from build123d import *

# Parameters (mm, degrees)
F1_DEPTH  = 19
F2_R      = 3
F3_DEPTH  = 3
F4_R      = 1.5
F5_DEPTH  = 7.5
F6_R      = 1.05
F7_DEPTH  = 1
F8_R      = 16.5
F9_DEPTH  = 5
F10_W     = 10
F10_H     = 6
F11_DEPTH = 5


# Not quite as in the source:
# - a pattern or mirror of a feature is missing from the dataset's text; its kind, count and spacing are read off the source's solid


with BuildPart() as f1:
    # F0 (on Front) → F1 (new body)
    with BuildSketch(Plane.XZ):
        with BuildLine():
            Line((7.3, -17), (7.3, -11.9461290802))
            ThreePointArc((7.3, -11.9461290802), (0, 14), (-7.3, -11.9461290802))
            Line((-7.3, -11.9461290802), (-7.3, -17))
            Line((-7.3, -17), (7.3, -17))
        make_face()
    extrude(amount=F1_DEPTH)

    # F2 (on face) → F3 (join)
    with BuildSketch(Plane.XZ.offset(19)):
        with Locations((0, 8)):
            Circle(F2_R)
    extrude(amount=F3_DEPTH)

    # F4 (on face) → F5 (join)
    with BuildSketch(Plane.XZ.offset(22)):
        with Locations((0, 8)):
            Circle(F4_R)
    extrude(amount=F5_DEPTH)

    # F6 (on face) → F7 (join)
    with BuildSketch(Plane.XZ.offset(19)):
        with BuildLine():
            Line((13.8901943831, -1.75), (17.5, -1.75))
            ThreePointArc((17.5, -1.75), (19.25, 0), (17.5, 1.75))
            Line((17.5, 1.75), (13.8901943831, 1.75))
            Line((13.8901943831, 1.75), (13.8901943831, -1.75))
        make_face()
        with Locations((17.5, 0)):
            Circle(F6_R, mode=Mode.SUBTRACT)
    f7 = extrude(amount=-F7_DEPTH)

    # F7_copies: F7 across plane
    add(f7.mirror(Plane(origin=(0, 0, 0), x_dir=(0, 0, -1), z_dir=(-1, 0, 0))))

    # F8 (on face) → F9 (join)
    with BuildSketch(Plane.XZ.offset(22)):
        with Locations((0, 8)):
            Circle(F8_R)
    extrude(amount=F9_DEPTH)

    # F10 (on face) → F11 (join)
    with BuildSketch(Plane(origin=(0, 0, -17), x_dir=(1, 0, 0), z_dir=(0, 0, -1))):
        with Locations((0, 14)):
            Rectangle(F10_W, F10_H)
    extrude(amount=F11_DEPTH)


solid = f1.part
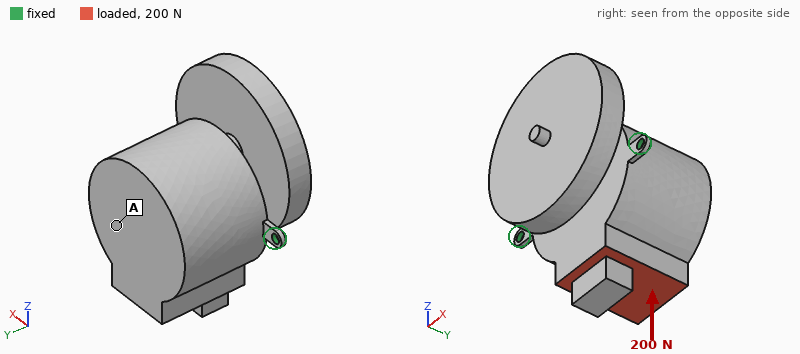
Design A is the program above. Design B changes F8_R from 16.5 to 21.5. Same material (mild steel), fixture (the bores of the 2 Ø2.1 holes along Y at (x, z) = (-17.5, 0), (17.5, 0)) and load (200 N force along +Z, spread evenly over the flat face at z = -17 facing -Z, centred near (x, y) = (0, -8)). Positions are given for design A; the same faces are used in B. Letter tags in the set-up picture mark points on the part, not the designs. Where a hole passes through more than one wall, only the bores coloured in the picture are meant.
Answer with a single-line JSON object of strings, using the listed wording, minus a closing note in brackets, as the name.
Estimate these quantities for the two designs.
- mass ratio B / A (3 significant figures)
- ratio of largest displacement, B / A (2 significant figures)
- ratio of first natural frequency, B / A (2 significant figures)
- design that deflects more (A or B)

{"mass ratio B / A": "1.17", "ratio of largest displacement, B / A": "1.2", "ratio of first natural frequency, B / A": "0.88", "design that deflects more": "B"}
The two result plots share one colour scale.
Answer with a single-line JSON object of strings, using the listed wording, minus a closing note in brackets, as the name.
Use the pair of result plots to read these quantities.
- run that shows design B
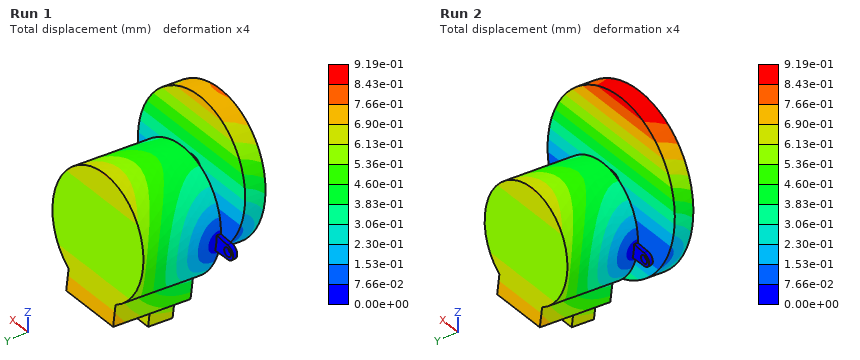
{"run that shows design B": "Run 2"}
